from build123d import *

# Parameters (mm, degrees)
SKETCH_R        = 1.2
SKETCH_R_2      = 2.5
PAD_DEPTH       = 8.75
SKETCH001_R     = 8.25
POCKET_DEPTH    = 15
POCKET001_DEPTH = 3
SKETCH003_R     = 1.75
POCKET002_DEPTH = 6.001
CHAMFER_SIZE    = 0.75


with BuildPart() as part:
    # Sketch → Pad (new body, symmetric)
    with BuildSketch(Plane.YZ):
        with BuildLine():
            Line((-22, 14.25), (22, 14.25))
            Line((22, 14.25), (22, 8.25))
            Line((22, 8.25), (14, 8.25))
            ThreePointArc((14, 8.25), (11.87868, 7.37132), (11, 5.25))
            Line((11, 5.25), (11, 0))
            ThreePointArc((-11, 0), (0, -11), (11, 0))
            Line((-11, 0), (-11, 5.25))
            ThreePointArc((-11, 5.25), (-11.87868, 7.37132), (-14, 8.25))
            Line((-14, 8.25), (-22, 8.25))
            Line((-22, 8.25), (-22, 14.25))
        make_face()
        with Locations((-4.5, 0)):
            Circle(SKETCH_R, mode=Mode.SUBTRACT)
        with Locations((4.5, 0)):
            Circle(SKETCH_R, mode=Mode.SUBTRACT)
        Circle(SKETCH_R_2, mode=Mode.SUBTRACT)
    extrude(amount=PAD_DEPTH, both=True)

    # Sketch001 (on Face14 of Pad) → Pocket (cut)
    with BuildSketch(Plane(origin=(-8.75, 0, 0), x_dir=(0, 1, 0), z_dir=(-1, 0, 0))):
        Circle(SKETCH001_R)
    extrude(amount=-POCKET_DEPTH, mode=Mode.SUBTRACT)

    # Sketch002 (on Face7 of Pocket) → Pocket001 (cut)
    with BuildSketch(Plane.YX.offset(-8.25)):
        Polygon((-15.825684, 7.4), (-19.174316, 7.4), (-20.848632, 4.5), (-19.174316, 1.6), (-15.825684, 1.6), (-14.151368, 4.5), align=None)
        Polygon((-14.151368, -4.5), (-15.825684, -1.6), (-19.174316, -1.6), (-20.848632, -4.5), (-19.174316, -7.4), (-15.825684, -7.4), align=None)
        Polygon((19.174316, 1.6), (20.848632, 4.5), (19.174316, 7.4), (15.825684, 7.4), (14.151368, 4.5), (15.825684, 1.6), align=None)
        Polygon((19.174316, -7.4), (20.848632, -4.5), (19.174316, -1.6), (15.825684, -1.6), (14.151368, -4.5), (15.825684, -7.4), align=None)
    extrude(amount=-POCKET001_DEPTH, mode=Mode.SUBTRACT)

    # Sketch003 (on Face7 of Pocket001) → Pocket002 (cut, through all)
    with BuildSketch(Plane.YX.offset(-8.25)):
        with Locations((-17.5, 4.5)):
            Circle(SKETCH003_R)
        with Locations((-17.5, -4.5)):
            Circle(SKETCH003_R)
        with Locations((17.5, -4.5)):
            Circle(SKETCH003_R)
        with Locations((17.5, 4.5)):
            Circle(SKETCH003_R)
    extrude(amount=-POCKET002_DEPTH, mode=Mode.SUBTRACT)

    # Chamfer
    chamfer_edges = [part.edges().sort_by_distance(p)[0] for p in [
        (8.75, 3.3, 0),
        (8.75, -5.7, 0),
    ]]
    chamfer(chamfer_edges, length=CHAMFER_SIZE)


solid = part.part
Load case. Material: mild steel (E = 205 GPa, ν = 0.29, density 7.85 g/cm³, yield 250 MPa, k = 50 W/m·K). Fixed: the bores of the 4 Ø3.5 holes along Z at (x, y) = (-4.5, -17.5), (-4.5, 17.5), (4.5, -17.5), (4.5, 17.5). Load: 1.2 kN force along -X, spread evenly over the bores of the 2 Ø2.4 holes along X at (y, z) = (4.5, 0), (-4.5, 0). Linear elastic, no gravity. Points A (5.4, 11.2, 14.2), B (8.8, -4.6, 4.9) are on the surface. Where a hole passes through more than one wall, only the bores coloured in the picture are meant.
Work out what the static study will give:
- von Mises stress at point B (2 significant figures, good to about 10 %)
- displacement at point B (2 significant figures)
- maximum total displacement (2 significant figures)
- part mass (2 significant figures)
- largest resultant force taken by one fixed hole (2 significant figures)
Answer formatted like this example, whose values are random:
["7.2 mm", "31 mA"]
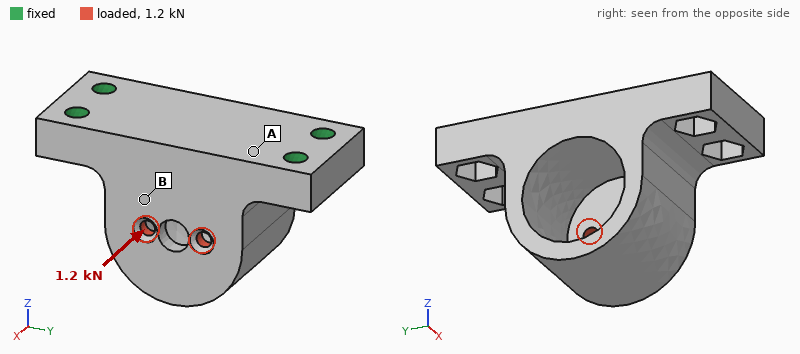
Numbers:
["61 MPa", "8.2 µm", "16 µm", "58 g", "880 N"]
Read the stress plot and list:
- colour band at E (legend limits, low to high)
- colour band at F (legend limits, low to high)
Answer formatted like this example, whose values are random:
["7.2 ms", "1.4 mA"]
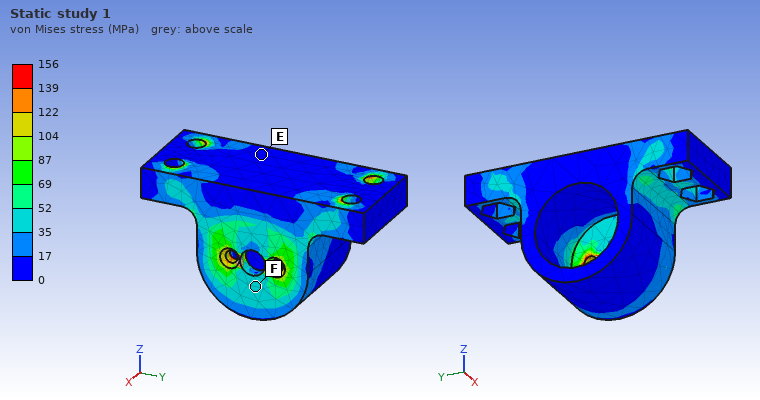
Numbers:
["0 to 17 MPa", "35 to 52 MPa"]
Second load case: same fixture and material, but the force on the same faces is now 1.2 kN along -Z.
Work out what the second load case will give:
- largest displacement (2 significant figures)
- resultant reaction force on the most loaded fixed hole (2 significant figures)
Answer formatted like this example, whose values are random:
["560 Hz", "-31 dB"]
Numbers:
["8.8 µm", "800 N"]
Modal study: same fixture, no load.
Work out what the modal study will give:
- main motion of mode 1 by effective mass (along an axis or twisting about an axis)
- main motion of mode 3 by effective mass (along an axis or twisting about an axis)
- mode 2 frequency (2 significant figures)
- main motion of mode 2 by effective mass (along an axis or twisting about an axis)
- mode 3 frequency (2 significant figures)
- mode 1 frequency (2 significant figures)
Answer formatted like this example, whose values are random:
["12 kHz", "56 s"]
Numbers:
["along X", "along Z", "15 kHz", "along Y", "18 kHz", "10 kHz"]
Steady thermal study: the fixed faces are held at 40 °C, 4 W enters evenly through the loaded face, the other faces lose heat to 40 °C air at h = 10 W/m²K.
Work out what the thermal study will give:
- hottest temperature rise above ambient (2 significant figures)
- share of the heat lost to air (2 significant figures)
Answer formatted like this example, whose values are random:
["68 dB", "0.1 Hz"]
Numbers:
["15 K", "5.1 %"]
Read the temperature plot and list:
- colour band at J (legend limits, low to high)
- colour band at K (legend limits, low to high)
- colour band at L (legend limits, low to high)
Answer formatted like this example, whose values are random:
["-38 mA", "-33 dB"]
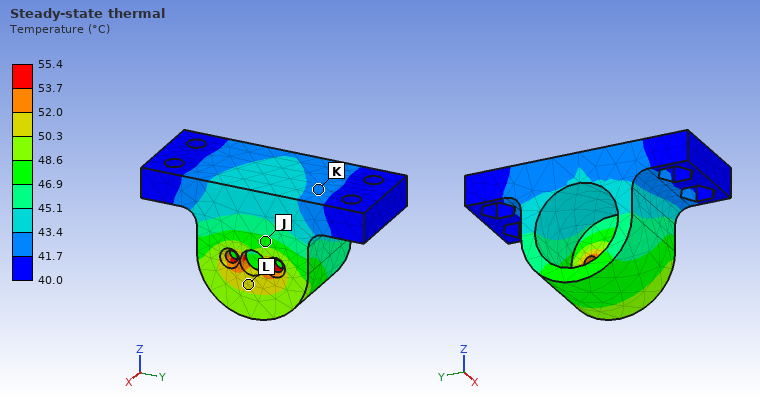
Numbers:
["46.9 to 48.6 °C", "41.7 to 43.4 °C", "50.3 to 52.0 °C"]
